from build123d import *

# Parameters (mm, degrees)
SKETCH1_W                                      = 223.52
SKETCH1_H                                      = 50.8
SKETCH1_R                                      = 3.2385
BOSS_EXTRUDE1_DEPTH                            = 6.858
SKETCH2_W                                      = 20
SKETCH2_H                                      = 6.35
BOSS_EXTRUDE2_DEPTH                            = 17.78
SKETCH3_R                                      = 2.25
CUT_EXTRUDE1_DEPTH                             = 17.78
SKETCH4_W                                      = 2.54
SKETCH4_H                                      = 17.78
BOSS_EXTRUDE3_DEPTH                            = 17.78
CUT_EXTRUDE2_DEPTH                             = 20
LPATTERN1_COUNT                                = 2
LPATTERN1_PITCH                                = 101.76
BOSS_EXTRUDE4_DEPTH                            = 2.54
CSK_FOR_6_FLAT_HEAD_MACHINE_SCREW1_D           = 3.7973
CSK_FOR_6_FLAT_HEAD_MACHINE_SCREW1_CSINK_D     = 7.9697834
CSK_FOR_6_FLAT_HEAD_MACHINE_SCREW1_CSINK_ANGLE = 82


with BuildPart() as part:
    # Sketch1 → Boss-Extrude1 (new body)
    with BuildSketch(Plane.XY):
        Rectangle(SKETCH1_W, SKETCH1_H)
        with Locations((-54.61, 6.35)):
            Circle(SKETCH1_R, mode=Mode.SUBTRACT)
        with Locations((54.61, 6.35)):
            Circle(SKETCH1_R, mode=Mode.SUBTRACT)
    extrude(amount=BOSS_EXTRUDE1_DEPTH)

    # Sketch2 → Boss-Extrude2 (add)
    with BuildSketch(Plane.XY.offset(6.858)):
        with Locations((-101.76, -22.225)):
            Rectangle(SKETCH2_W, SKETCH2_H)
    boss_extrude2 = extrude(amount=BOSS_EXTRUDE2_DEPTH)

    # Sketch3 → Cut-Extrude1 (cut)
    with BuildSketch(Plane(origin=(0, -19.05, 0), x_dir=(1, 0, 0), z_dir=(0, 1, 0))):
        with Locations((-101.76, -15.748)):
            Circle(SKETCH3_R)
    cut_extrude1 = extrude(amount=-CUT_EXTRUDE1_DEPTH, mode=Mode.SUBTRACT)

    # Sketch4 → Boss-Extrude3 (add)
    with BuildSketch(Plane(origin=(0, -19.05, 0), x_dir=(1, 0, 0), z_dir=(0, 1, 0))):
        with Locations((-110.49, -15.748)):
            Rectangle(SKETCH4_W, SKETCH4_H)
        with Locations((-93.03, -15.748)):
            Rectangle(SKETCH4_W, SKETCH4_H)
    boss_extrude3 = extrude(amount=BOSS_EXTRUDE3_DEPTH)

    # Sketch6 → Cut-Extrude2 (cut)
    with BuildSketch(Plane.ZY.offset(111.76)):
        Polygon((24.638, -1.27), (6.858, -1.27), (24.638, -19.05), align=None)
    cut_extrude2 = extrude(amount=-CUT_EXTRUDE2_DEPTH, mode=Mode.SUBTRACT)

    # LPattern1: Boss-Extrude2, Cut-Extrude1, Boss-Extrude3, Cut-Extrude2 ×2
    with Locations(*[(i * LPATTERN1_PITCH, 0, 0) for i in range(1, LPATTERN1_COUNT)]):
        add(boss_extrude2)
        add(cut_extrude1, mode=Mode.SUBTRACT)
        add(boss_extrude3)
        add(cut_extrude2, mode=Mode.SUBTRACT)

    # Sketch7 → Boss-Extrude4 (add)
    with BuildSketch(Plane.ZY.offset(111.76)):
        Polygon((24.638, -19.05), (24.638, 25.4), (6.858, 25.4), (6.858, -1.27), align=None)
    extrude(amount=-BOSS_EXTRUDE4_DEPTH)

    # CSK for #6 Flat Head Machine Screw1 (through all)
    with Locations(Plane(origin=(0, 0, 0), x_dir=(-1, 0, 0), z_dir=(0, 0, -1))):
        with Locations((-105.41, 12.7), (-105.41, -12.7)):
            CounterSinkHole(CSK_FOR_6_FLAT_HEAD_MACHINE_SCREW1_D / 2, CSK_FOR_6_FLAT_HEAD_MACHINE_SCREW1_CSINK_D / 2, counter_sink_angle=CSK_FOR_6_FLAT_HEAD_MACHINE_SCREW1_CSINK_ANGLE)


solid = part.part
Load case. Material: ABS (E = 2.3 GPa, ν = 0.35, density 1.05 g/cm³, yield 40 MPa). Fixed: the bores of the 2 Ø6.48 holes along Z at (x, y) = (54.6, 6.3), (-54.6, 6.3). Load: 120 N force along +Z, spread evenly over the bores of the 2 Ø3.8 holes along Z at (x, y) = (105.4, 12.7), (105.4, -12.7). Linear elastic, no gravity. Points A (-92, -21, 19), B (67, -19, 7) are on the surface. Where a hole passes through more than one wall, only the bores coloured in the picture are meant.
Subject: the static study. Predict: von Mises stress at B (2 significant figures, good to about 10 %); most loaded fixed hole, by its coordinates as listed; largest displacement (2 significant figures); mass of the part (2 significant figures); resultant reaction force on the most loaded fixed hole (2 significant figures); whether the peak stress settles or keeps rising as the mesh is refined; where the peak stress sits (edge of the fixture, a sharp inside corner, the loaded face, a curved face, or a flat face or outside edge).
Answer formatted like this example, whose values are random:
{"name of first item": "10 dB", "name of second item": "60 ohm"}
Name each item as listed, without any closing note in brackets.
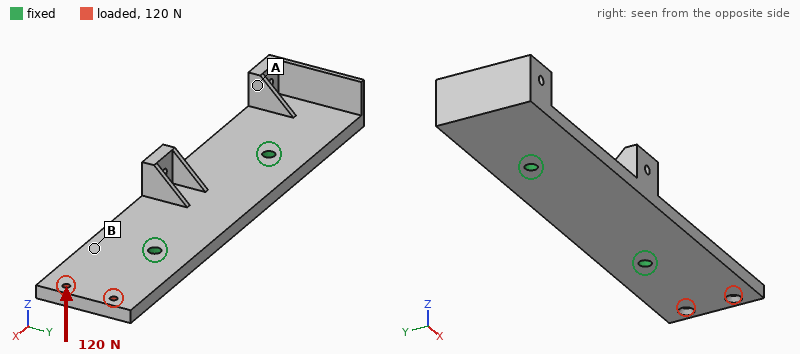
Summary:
{"von Mises stress at B": "8.9 MPa", "most loaded fixed hole, by its coordinates as listed": "(54.6, 6.3)", "largest displacement": "2.3 mm", "mass of the part": "89 g", "resultant reaction force on the most loaded fixed hole": "130 N", "whether the peak stress settles or keeps rising as the mesh is refined": "keeps rising", "where the peak stress sits": "edge of the fixture"}
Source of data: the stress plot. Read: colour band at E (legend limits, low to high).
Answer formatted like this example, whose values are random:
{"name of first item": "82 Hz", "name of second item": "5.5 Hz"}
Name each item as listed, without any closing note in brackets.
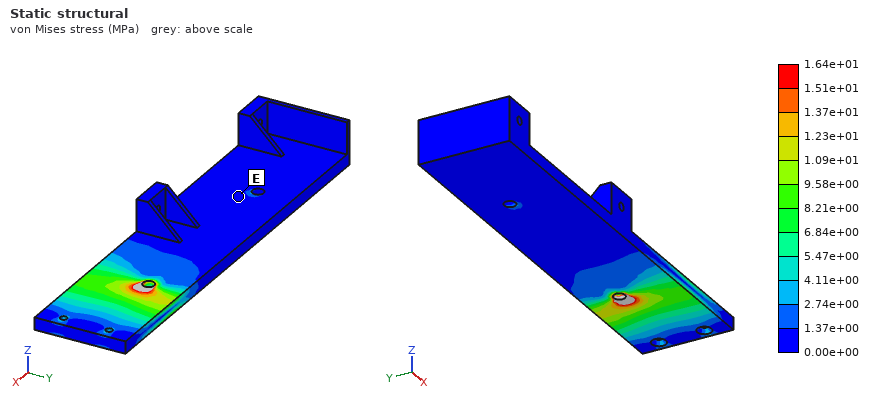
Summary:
{"colour band at E": "0.00e+00 to 1.37e+00 MPa"}
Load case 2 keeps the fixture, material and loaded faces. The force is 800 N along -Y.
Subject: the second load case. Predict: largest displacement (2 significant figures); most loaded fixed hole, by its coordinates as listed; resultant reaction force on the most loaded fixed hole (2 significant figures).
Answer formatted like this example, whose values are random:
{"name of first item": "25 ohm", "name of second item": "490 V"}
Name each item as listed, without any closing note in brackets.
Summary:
{"largest displacement": "1.1 mm", "most loaded fixed hole, by its coordinates as listed": "(54.6, 6.3)", "resultant reaction force on the most loaded fixed hole": "1.2 kN"}
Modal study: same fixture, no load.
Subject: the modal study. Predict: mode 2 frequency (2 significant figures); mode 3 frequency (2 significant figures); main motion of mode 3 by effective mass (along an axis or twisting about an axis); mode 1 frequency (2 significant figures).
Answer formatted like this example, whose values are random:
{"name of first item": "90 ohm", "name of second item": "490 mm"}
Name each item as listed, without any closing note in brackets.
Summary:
{"mode 2 frequency": "460 Hz", "mode 3 frequency": "660 Hz", "main motion of mode 3 by effective mass": "along Z", "mode 1 frequency": "350 Hz"}
